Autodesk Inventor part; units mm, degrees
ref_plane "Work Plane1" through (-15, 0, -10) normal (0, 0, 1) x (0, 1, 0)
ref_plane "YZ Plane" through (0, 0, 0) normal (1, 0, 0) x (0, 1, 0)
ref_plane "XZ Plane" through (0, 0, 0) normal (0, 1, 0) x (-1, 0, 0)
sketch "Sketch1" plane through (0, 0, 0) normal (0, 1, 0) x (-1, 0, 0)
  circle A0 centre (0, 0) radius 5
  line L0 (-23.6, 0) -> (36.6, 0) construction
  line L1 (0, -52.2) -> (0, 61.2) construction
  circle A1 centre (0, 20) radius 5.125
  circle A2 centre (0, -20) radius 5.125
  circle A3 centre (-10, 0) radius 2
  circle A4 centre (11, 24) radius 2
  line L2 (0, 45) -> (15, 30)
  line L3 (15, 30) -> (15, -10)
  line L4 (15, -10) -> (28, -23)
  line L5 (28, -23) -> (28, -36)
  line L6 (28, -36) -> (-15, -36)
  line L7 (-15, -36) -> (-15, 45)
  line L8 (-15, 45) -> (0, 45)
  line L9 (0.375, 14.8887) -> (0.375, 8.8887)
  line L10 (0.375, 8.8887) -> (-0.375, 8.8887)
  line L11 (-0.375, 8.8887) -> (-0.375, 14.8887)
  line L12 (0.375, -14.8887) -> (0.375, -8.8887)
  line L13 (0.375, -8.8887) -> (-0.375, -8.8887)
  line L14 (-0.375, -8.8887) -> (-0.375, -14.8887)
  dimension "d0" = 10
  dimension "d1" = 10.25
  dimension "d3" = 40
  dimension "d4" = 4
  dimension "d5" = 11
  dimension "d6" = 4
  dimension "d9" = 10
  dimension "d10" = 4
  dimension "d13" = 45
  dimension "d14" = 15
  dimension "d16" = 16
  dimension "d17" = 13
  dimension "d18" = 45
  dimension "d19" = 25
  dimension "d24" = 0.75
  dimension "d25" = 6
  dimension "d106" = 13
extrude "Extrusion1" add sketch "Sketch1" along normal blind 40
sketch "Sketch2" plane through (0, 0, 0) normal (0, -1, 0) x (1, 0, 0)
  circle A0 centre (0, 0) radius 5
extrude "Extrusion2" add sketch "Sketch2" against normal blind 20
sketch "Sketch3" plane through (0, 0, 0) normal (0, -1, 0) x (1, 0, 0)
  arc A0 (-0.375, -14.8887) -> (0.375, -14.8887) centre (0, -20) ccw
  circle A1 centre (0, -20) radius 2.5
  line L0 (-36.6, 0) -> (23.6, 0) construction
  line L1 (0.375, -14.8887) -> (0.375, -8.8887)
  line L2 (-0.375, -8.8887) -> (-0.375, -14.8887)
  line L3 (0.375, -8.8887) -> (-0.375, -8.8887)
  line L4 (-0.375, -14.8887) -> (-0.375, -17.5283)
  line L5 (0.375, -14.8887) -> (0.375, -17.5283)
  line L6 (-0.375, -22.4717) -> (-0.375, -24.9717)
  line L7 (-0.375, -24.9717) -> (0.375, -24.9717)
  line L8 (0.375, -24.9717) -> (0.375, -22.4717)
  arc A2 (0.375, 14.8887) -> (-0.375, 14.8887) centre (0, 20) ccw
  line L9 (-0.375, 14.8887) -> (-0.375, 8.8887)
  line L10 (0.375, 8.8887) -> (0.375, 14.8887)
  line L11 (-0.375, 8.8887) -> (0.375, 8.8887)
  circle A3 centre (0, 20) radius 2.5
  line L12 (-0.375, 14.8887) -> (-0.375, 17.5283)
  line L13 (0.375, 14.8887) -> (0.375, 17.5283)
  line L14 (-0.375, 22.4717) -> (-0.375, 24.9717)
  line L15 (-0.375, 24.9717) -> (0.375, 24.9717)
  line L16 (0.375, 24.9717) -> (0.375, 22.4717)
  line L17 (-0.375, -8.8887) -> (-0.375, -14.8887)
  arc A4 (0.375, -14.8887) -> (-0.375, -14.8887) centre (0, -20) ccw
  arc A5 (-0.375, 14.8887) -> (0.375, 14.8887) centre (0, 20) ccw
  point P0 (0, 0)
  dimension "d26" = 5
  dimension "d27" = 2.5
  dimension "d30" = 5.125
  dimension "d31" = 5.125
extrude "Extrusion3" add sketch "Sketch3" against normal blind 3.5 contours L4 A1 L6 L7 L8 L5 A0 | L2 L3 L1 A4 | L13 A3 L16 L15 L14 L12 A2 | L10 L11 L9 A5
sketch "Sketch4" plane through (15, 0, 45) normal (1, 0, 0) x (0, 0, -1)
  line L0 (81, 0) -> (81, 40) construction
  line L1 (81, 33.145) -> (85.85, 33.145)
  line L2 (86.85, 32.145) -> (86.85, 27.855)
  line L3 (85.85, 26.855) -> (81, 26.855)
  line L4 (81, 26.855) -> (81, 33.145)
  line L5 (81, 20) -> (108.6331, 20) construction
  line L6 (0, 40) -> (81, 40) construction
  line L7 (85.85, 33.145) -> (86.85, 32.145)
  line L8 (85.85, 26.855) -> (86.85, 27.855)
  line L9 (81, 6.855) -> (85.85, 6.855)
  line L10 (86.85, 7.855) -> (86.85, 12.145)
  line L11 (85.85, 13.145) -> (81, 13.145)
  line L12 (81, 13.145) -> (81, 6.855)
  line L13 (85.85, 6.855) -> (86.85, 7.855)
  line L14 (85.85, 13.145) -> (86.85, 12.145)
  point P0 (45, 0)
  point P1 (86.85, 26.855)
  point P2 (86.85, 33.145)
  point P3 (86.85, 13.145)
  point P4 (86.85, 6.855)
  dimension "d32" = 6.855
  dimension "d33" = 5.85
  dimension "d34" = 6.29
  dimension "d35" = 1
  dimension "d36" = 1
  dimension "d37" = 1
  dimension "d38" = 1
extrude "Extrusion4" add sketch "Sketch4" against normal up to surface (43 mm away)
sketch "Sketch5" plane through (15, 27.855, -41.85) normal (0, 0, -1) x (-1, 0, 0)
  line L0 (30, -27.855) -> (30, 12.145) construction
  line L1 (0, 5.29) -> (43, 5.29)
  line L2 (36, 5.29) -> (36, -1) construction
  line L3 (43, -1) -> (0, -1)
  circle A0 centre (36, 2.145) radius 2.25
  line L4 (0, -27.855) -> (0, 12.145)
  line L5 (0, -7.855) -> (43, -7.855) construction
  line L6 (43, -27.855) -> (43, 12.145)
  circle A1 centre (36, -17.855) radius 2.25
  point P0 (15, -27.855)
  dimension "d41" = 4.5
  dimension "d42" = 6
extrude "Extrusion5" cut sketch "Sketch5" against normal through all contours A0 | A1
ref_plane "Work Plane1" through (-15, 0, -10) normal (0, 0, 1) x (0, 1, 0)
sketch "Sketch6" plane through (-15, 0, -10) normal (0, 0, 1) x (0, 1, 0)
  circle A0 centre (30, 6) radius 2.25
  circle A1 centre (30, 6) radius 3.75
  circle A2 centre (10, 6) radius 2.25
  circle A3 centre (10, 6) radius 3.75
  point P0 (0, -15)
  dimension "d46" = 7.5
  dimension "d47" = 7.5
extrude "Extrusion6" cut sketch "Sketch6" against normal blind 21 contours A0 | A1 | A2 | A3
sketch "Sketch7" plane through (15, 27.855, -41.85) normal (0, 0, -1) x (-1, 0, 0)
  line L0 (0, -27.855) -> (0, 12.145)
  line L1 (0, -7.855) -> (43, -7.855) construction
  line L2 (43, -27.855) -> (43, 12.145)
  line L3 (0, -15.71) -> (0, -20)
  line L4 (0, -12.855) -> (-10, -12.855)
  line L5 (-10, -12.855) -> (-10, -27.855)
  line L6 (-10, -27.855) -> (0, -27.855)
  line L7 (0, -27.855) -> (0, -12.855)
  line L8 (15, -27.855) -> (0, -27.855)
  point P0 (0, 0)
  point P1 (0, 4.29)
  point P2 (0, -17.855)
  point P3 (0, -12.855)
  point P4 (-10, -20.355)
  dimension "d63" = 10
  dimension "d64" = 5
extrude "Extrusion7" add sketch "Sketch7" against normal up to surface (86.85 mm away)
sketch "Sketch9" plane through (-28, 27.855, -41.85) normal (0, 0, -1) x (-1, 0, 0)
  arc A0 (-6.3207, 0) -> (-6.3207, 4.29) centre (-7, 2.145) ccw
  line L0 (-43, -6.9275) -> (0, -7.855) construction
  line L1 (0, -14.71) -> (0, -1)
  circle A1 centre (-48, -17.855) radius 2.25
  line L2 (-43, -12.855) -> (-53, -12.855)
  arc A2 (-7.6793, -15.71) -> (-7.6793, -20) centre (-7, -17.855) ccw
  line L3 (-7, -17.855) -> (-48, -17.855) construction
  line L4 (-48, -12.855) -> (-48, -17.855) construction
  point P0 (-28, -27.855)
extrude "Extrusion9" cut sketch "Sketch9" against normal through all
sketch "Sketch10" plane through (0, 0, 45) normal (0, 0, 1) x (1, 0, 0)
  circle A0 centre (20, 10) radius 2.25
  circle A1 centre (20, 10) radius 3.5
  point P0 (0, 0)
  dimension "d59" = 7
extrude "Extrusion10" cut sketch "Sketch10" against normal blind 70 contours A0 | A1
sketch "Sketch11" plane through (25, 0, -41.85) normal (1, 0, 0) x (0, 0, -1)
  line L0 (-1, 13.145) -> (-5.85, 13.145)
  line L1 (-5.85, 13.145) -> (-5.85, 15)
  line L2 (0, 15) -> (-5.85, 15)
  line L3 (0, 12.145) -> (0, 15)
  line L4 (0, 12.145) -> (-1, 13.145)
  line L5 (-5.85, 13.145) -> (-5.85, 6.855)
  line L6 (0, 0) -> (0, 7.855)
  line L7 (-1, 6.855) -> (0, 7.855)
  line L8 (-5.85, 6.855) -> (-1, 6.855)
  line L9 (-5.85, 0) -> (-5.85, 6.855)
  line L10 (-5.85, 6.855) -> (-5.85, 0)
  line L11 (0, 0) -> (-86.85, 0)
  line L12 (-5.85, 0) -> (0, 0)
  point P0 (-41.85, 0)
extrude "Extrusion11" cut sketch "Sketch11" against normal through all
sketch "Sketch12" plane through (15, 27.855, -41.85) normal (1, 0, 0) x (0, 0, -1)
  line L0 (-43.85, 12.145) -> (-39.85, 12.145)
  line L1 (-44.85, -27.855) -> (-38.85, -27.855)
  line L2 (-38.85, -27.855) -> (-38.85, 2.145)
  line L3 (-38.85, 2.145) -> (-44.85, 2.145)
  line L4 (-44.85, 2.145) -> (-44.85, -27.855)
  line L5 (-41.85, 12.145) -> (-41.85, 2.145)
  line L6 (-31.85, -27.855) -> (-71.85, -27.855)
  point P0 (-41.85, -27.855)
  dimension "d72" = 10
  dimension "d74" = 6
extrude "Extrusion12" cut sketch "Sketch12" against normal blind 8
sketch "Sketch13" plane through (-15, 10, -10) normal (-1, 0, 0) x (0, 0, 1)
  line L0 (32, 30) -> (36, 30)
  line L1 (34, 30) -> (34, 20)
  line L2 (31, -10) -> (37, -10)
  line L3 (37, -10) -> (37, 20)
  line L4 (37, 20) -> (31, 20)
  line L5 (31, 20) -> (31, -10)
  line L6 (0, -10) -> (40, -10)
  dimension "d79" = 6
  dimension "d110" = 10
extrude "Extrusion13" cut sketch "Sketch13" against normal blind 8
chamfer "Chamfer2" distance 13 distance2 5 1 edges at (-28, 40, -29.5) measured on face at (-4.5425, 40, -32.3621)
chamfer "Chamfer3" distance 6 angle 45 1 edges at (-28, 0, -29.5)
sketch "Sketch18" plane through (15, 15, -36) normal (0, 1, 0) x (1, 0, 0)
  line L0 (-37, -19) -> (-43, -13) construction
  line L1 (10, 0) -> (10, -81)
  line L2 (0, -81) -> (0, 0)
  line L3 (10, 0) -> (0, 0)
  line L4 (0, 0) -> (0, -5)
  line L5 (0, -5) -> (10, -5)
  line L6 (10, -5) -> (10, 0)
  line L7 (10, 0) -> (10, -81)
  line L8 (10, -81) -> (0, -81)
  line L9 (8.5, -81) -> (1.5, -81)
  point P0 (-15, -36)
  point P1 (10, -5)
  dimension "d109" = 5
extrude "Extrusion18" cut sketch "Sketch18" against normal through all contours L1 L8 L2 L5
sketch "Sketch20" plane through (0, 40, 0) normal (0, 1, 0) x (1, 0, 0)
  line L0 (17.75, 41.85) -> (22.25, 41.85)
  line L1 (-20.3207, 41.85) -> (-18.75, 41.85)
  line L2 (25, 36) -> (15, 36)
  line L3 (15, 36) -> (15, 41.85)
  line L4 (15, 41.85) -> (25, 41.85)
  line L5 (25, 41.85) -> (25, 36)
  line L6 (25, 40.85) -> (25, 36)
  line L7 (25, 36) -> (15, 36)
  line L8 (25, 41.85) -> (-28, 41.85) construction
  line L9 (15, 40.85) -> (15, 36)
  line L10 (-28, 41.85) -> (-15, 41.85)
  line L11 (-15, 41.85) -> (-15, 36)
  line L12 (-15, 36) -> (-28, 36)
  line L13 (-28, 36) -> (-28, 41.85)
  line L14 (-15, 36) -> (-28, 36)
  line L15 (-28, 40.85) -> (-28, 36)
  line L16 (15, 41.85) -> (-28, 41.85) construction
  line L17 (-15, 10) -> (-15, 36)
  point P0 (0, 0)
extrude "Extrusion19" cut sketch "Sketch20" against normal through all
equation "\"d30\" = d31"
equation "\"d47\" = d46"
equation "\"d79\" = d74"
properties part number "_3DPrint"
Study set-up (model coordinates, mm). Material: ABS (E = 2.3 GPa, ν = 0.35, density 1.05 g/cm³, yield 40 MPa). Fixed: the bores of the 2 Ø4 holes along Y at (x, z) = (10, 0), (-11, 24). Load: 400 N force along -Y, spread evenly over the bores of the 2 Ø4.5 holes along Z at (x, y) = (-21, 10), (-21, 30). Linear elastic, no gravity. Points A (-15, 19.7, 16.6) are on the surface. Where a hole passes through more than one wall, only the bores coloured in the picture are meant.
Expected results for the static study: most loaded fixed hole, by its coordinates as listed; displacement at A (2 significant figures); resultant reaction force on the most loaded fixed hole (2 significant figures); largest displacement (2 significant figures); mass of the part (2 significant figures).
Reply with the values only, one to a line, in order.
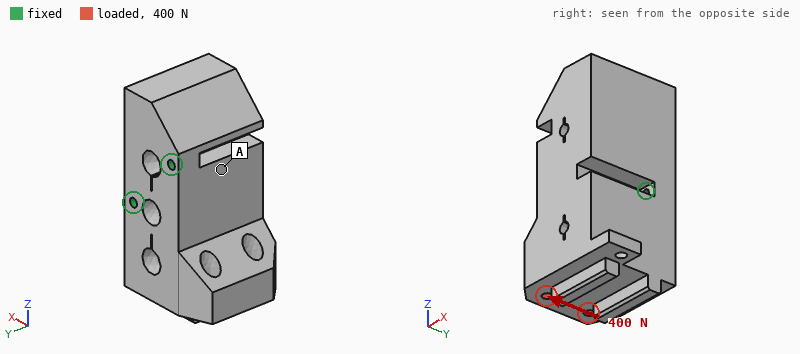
(10, 0)
0.26 mm
370 N
1.1 mm
97 g
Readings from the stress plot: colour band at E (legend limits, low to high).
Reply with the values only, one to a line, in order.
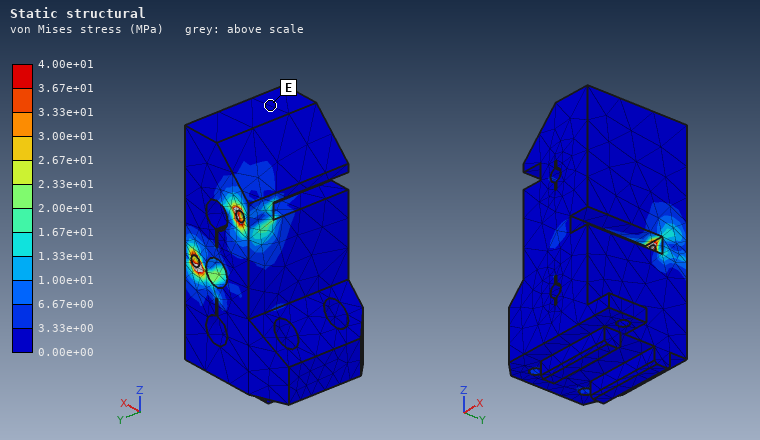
0.00e+00 to 3.33e+00 MPa
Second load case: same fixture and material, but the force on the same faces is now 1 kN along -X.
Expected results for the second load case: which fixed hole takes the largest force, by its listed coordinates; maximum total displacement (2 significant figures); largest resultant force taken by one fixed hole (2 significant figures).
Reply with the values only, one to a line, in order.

(10, 0)
0.90 mm
1.8 kN
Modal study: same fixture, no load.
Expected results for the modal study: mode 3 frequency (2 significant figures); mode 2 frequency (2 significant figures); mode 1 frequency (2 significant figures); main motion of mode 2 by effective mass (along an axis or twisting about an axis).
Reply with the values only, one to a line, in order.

1900 Hz
1400 Hz
600 Hz
along X
